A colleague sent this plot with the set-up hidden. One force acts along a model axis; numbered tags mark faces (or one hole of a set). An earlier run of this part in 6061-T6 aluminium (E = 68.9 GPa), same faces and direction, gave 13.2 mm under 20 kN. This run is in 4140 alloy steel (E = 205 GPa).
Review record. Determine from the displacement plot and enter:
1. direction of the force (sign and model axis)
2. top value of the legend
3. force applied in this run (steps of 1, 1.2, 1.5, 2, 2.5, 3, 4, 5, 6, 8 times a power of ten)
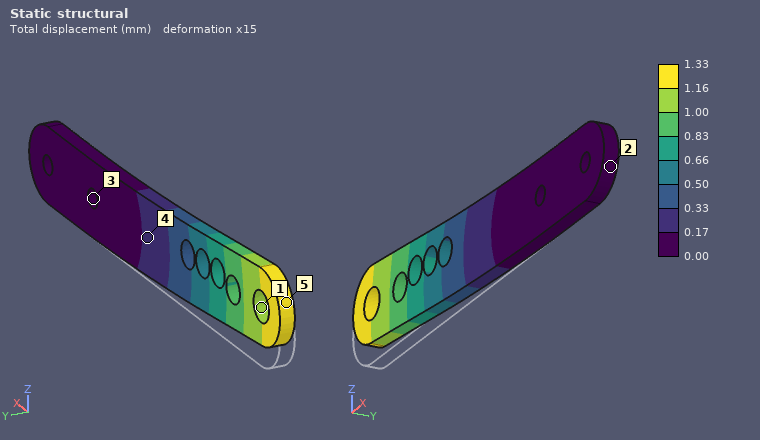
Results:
+Z
1.33 mm
6 kN
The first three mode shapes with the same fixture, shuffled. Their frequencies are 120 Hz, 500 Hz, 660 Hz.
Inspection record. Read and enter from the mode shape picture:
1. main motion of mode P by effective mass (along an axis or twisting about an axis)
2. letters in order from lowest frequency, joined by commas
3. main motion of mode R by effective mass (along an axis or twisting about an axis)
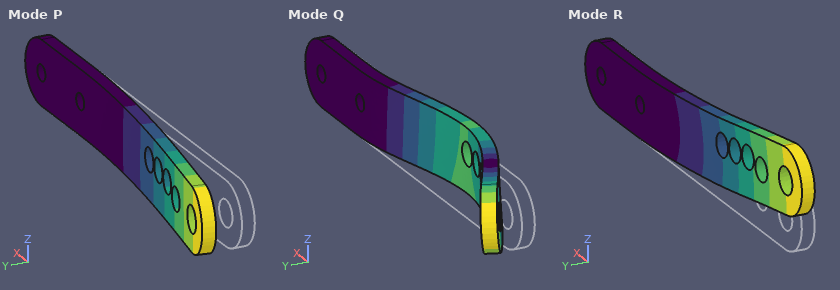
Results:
along Y
P, R, Q
along Z
